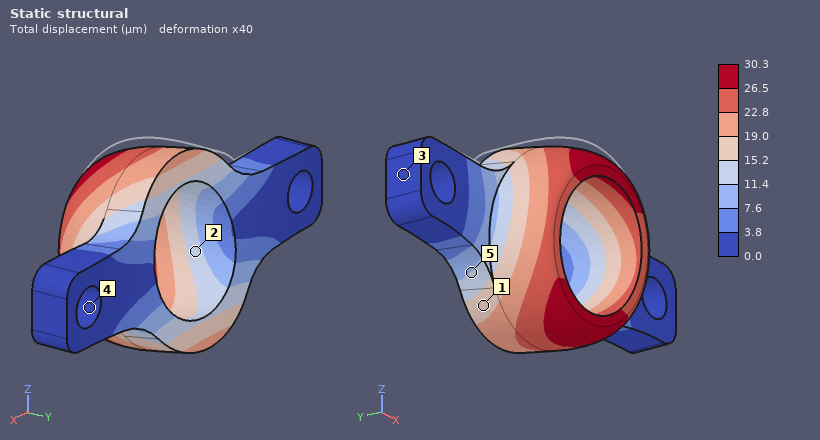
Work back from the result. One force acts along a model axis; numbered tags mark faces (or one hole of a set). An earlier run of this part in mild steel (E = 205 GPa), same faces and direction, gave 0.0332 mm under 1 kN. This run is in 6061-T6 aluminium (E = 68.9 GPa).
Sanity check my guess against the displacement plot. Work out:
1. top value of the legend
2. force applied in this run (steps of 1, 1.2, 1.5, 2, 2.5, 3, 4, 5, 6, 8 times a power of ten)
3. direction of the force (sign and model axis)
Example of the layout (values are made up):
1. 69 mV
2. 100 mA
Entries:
1. 30.3 µm
2. 300 N
3. -Z
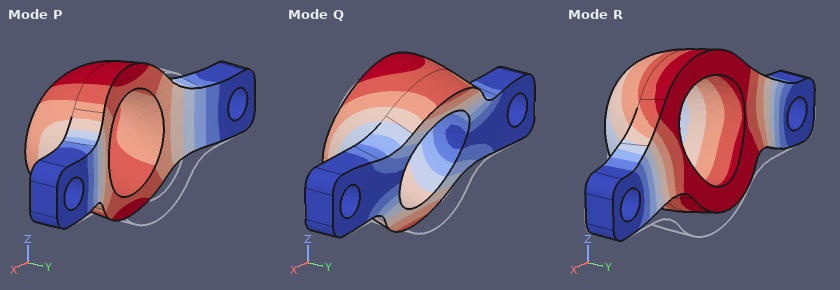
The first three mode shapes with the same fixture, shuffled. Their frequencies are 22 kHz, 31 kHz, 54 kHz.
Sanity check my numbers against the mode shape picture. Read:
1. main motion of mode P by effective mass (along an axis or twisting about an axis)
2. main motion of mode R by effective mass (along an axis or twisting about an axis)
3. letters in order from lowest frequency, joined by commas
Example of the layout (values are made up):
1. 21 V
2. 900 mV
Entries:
1. along Y
2. along Z
3. Q, P, R
